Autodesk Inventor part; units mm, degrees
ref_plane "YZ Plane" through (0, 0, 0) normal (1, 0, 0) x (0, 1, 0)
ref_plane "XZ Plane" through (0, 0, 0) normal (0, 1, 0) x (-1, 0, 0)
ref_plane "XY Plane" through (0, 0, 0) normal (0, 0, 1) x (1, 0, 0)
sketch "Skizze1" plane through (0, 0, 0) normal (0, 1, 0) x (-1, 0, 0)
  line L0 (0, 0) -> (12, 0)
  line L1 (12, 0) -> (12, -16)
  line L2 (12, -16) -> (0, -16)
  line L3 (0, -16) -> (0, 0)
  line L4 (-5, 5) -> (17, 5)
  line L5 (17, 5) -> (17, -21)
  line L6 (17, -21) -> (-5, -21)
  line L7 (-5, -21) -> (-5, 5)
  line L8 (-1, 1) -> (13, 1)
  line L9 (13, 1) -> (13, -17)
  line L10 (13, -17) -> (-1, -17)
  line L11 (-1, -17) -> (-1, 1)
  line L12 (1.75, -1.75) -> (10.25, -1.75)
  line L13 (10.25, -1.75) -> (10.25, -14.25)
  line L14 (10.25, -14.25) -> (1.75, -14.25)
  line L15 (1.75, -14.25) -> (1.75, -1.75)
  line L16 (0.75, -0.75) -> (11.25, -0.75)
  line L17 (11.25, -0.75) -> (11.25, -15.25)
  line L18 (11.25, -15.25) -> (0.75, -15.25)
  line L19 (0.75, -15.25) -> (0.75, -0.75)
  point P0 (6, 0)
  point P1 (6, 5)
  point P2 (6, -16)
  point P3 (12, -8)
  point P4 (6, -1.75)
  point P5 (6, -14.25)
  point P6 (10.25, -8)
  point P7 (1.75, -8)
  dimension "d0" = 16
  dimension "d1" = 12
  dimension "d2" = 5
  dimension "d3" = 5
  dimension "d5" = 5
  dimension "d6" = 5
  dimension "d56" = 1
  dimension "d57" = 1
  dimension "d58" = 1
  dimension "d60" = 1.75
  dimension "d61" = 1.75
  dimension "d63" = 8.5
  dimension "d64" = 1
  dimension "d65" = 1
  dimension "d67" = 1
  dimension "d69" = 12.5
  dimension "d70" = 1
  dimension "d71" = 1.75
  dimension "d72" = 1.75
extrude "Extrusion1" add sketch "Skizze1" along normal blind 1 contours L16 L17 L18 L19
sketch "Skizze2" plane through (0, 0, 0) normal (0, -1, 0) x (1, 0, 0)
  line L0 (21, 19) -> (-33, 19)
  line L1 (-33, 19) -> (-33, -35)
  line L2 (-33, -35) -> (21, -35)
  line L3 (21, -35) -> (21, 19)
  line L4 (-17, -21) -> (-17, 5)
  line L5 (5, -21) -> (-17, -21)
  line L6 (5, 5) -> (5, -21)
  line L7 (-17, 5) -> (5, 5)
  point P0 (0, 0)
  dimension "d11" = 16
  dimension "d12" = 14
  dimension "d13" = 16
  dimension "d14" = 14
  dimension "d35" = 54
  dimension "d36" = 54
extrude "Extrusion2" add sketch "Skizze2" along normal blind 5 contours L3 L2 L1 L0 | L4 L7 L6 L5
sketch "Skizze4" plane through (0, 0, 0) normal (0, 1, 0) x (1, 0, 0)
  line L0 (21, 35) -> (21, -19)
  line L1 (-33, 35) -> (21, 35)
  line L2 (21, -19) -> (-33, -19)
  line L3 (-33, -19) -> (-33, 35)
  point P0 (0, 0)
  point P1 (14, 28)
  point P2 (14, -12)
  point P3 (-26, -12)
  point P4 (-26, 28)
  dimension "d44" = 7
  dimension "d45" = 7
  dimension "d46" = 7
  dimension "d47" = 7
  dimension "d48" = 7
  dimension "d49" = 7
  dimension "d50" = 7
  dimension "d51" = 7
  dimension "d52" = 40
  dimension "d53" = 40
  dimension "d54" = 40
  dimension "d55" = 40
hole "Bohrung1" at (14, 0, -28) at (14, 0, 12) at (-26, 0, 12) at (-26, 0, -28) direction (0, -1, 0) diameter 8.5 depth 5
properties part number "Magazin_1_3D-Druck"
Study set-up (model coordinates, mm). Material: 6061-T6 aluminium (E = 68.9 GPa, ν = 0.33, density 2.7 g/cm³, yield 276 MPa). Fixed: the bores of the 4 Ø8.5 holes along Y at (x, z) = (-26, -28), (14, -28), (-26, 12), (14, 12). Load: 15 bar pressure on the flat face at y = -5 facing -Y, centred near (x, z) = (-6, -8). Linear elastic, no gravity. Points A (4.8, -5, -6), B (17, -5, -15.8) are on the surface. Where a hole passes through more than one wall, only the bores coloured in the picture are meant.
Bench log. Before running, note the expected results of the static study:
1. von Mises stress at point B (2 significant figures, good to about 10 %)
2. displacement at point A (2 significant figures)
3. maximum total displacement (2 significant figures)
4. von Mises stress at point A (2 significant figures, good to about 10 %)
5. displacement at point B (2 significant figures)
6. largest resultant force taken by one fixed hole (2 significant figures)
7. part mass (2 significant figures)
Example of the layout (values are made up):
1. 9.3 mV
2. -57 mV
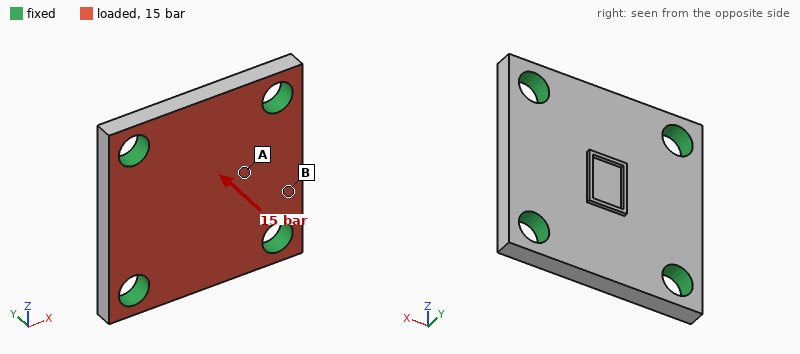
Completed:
1. 8.3 MPa
2. 17 µm
3. 22 µm
4. 18 MPa
5. 6.5 µm
6. 1.0 kN
7. 36 g
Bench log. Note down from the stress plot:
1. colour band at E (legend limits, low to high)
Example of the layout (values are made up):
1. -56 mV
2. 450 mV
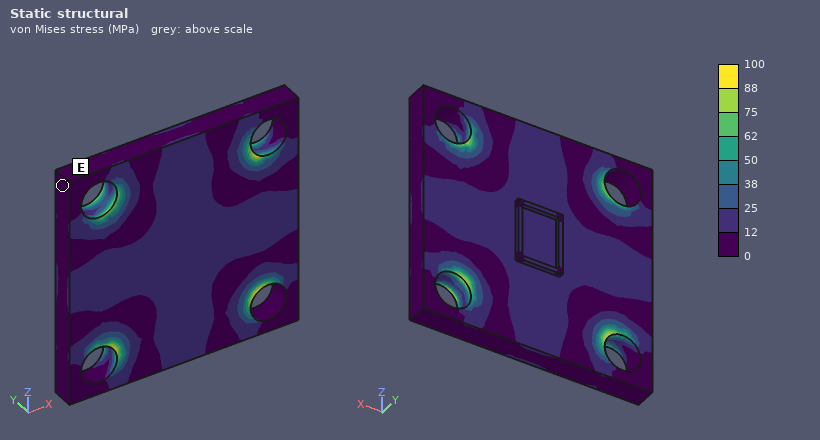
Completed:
1. 0 to 12 MPa
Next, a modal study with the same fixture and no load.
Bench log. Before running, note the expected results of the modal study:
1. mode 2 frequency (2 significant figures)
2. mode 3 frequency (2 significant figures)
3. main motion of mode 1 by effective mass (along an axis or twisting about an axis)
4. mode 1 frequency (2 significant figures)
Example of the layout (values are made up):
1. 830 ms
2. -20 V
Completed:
1. 21 kHz
2. 21 kHz
3. along Y
4. 14 kHz
